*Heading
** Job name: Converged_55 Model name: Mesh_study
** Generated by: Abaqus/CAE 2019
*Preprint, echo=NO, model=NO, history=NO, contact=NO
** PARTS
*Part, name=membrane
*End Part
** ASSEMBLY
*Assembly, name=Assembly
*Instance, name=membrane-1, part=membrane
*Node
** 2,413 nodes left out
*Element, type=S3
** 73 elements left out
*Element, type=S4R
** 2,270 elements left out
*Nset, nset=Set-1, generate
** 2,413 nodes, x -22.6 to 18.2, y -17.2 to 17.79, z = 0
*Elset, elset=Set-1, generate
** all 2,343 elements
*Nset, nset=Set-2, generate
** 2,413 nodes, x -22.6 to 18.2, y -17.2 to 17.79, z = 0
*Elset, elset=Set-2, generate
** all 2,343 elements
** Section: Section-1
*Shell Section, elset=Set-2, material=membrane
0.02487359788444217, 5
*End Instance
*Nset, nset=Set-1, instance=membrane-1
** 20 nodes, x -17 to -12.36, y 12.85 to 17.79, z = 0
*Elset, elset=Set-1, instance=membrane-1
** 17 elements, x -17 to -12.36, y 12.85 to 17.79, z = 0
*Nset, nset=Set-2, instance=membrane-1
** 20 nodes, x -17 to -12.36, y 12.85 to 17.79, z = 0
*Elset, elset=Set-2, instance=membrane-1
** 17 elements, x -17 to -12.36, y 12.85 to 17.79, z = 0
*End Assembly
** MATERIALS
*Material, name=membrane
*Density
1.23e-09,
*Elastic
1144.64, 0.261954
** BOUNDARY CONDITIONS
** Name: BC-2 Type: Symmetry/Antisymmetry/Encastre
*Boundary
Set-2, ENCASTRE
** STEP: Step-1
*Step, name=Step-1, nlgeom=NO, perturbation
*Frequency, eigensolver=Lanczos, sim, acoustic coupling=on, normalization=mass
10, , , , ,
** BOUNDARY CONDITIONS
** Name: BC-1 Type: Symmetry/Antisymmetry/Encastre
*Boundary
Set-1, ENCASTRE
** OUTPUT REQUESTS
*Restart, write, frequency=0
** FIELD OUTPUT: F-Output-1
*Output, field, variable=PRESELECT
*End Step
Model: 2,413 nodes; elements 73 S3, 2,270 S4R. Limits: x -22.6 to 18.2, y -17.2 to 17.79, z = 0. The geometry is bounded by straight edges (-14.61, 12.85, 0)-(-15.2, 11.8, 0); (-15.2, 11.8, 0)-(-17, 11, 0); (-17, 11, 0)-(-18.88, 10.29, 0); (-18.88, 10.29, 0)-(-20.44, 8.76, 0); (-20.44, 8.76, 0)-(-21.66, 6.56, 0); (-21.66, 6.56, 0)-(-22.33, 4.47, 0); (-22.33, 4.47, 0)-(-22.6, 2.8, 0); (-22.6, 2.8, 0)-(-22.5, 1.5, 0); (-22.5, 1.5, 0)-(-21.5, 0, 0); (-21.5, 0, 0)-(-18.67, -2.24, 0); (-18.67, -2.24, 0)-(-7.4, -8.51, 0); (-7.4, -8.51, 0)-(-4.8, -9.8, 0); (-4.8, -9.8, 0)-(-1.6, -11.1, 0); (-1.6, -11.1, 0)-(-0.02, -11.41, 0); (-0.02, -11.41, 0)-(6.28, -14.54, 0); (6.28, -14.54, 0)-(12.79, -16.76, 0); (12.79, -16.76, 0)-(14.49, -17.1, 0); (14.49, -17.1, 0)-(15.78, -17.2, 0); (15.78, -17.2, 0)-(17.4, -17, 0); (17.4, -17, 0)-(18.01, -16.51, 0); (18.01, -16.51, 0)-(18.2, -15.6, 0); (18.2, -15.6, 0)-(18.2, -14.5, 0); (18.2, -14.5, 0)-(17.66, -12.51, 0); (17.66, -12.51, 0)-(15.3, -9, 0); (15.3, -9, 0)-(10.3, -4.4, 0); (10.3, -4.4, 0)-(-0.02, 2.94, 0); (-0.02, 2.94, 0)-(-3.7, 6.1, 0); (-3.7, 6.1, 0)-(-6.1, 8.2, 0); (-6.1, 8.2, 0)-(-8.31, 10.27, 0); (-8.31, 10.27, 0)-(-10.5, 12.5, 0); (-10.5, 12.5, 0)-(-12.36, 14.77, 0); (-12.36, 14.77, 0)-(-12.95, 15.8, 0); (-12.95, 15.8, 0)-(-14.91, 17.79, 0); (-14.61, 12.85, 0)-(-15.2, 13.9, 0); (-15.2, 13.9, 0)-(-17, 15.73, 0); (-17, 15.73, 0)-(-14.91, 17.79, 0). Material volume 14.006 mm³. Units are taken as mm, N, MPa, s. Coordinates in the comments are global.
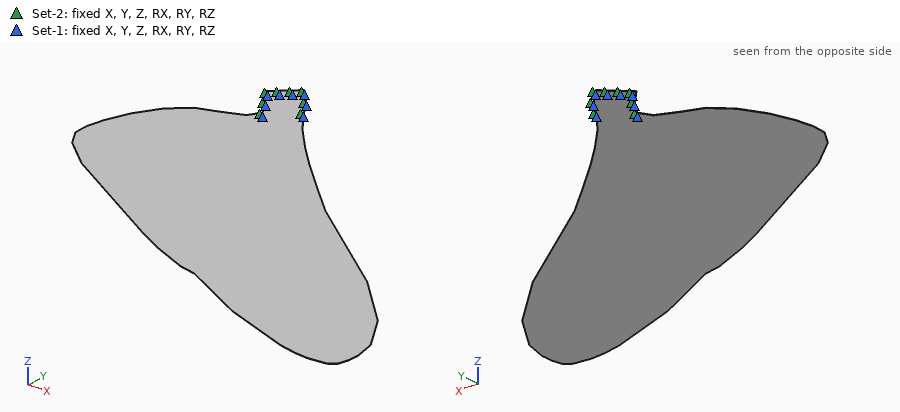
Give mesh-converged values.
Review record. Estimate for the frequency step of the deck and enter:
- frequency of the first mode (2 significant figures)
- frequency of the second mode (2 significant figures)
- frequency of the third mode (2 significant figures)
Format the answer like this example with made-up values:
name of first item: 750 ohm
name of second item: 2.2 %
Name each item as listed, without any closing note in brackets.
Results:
frequency of the first mode: 2.0 Hz
frequency of the second mode: 8.3 Hz
frequency of the third mode: 16 Hz
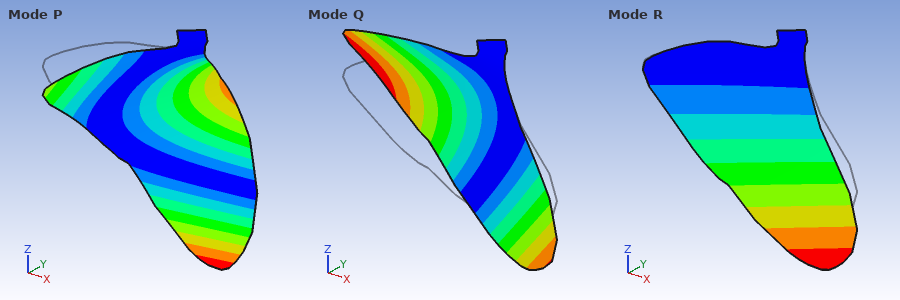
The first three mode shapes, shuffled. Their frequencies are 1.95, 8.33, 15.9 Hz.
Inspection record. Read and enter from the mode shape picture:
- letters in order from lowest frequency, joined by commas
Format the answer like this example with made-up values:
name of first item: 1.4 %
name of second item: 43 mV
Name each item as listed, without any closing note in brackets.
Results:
letters in order from lowest frequency, joined by commas: R, Q, P
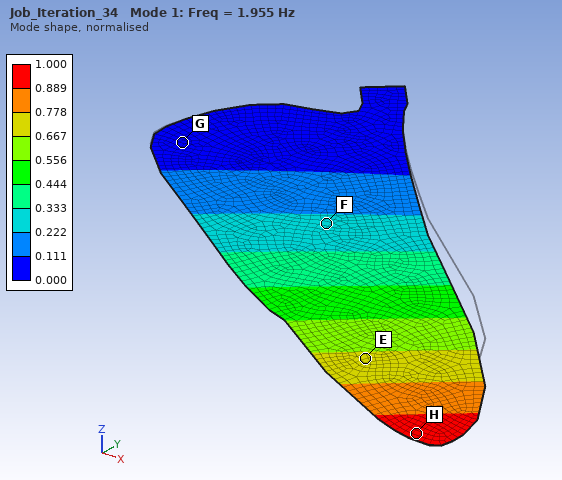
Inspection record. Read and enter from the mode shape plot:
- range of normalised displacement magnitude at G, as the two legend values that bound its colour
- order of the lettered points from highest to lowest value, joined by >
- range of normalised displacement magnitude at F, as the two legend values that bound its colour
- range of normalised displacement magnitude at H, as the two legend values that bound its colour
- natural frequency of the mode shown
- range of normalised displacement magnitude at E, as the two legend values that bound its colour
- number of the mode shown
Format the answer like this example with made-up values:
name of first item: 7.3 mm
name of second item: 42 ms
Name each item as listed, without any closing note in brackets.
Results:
range of normalised displacement magnitude at G, as the two legend values that bound its colour: 0.000 to 0.111
order of the lettered points from highest to lowest value, joined by >: H > E > F > G
range of normalised displacement magnitude at F, as the two legend values that bound its colour: 0.222 to 0.333
range of normalised displacement magnitude at H, as the two legend values that bound its colour: 0.889 to 1.000
natural frequency of the mode shown: 1.955 Hz
range of normalised displacement magnitude at E, as the two legend values that bound its colour: 0.667 to 0.778
number of the mode shown: 1
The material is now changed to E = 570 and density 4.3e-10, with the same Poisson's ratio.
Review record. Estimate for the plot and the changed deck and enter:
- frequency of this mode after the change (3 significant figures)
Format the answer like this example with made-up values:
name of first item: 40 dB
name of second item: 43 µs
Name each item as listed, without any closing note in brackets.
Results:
frequency of this mode after the change: 2.33 Hz
